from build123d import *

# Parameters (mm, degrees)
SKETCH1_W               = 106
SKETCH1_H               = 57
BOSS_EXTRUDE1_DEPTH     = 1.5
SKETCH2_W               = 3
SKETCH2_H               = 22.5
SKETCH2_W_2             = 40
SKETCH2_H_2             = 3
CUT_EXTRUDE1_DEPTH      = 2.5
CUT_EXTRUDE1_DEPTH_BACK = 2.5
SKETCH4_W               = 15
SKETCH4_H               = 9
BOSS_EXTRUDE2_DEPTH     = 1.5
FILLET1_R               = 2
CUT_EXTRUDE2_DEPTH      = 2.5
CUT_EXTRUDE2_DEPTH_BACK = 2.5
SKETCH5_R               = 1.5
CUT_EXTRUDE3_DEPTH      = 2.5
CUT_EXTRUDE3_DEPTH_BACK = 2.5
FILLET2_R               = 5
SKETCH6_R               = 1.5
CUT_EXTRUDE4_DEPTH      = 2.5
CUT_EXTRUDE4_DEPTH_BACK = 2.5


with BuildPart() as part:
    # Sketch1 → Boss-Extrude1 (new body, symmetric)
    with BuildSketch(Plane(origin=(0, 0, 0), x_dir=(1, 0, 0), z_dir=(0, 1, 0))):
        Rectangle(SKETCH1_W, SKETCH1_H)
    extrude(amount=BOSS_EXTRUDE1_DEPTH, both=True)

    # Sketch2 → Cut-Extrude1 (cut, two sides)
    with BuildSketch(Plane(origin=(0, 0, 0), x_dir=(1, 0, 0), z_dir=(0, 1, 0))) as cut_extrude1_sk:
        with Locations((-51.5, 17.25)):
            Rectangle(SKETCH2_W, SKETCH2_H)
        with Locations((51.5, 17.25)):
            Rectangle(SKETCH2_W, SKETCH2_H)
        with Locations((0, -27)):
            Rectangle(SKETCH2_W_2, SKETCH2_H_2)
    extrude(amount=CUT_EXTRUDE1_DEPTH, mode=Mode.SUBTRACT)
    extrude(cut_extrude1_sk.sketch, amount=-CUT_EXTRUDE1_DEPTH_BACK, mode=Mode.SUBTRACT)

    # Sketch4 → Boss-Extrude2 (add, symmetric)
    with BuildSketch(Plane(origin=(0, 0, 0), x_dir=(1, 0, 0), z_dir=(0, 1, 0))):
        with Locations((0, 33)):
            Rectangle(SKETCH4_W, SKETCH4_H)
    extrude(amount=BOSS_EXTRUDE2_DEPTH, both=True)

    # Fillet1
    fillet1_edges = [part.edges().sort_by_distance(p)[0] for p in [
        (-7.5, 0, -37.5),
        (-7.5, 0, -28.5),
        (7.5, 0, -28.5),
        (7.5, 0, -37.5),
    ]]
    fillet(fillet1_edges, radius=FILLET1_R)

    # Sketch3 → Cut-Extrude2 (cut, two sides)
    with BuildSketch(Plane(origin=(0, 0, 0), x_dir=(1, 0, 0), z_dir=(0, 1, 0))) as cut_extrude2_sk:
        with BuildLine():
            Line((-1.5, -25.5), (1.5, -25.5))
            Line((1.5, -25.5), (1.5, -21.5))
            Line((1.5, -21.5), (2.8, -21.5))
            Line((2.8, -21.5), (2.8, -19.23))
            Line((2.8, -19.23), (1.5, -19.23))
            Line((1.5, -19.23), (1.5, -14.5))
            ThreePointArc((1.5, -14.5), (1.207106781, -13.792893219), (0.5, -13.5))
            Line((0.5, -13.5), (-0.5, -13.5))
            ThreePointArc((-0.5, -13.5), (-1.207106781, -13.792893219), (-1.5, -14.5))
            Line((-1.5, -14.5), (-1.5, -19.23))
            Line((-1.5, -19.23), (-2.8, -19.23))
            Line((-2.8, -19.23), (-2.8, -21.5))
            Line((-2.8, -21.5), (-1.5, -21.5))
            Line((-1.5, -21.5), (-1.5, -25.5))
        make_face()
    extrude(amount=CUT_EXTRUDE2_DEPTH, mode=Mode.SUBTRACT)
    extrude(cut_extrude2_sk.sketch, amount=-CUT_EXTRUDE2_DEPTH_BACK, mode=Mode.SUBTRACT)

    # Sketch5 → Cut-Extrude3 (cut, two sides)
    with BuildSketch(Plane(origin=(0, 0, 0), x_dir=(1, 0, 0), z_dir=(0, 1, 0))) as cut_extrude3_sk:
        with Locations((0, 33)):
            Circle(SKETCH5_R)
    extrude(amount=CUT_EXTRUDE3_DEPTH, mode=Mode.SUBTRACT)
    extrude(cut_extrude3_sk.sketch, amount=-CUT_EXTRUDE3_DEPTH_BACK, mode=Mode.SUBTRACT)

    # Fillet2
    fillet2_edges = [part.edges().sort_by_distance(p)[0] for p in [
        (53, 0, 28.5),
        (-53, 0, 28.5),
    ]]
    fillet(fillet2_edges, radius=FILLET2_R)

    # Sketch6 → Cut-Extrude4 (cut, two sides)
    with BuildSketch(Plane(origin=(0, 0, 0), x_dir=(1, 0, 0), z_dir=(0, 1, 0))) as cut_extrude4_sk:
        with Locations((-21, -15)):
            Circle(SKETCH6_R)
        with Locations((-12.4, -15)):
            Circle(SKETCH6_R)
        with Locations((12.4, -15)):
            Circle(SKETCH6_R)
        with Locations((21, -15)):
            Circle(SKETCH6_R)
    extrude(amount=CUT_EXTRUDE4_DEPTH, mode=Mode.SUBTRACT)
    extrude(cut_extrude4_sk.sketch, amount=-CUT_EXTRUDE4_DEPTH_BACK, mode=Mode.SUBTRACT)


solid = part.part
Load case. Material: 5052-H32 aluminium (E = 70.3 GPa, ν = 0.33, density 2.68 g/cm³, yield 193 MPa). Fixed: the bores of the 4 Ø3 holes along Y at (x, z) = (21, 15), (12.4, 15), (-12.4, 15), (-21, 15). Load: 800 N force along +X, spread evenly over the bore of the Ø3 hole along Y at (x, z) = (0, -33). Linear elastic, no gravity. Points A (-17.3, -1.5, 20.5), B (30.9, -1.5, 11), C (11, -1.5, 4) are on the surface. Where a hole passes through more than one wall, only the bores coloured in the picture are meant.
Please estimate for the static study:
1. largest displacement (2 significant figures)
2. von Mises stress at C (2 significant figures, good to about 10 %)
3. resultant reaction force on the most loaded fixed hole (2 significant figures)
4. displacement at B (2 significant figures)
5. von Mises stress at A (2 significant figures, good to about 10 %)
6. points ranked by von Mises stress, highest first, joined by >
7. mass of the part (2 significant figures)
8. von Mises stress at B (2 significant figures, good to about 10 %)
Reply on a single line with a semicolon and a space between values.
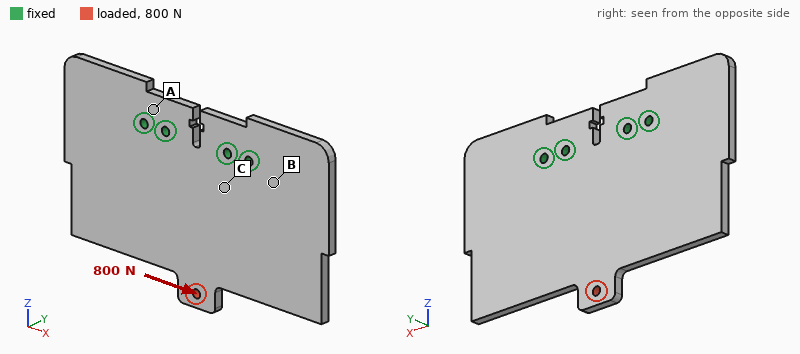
29 µm; 13 MPa; 810 N; 5.8 µm; 7.3 MPa; C > A > B; 47 g; 4.6 MPa
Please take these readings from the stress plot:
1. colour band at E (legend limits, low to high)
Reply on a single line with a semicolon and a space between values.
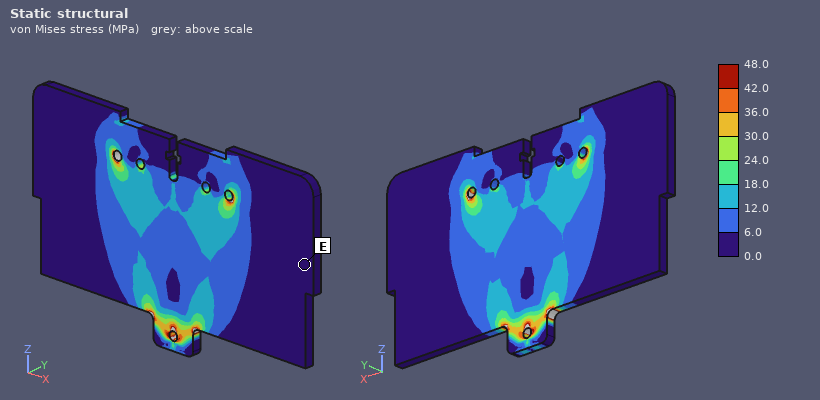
0.0 to 6.0 MPa
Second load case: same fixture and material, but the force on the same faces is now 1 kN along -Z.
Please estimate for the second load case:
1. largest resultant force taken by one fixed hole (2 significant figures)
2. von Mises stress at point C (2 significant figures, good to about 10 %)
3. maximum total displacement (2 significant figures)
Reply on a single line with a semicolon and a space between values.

270 N; 7.9 MPa; 11 µm
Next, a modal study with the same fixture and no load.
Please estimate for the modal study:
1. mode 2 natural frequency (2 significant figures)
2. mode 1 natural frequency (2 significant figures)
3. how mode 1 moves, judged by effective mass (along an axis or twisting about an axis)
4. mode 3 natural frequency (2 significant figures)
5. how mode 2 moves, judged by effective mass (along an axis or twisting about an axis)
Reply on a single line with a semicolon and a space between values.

1400 Hz; 1100 Hz; along Y; 2000 Hz; twisting about Z
